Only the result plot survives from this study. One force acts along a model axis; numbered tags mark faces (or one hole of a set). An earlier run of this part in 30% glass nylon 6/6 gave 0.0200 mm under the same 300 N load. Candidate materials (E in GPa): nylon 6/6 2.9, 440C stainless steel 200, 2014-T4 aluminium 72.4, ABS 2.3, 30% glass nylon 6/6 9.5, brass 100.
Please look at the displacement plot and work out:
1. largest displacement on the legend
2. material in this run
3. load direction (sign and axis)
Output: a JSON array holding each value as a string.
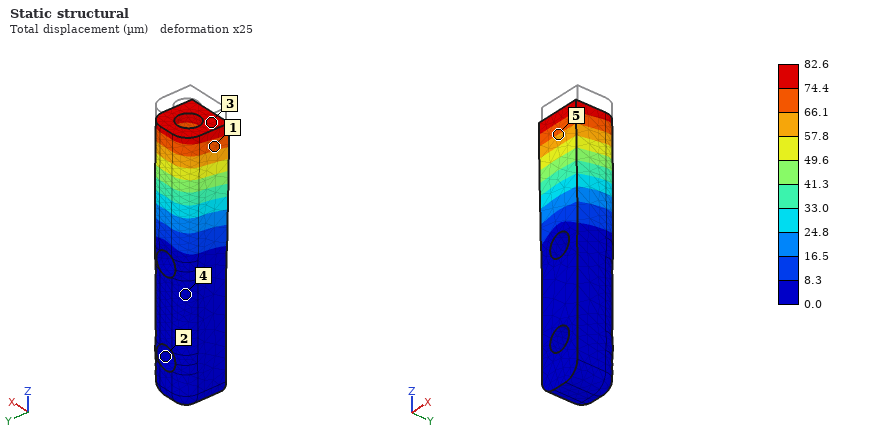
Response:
["82.6 µm", "ABS", "-Z"]
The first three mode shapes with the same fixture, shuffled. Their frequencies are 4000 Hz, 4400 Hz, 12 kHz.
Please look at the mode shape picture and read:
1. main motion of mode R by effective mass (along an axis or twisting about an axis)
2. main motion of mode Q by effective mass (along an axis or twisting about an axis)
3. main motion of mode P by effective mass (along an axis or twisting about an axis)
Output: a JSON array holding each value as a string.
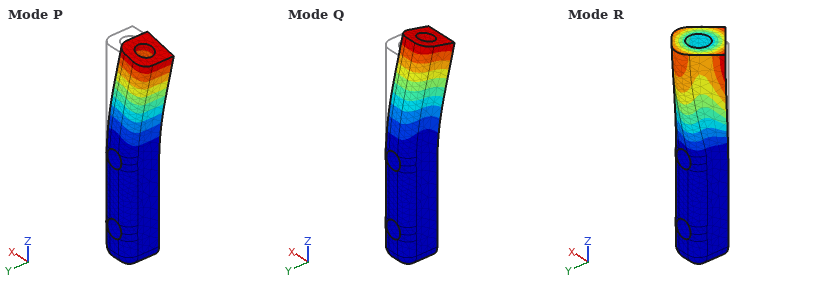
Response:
["twisting about Z", "along Y", "along X"]
